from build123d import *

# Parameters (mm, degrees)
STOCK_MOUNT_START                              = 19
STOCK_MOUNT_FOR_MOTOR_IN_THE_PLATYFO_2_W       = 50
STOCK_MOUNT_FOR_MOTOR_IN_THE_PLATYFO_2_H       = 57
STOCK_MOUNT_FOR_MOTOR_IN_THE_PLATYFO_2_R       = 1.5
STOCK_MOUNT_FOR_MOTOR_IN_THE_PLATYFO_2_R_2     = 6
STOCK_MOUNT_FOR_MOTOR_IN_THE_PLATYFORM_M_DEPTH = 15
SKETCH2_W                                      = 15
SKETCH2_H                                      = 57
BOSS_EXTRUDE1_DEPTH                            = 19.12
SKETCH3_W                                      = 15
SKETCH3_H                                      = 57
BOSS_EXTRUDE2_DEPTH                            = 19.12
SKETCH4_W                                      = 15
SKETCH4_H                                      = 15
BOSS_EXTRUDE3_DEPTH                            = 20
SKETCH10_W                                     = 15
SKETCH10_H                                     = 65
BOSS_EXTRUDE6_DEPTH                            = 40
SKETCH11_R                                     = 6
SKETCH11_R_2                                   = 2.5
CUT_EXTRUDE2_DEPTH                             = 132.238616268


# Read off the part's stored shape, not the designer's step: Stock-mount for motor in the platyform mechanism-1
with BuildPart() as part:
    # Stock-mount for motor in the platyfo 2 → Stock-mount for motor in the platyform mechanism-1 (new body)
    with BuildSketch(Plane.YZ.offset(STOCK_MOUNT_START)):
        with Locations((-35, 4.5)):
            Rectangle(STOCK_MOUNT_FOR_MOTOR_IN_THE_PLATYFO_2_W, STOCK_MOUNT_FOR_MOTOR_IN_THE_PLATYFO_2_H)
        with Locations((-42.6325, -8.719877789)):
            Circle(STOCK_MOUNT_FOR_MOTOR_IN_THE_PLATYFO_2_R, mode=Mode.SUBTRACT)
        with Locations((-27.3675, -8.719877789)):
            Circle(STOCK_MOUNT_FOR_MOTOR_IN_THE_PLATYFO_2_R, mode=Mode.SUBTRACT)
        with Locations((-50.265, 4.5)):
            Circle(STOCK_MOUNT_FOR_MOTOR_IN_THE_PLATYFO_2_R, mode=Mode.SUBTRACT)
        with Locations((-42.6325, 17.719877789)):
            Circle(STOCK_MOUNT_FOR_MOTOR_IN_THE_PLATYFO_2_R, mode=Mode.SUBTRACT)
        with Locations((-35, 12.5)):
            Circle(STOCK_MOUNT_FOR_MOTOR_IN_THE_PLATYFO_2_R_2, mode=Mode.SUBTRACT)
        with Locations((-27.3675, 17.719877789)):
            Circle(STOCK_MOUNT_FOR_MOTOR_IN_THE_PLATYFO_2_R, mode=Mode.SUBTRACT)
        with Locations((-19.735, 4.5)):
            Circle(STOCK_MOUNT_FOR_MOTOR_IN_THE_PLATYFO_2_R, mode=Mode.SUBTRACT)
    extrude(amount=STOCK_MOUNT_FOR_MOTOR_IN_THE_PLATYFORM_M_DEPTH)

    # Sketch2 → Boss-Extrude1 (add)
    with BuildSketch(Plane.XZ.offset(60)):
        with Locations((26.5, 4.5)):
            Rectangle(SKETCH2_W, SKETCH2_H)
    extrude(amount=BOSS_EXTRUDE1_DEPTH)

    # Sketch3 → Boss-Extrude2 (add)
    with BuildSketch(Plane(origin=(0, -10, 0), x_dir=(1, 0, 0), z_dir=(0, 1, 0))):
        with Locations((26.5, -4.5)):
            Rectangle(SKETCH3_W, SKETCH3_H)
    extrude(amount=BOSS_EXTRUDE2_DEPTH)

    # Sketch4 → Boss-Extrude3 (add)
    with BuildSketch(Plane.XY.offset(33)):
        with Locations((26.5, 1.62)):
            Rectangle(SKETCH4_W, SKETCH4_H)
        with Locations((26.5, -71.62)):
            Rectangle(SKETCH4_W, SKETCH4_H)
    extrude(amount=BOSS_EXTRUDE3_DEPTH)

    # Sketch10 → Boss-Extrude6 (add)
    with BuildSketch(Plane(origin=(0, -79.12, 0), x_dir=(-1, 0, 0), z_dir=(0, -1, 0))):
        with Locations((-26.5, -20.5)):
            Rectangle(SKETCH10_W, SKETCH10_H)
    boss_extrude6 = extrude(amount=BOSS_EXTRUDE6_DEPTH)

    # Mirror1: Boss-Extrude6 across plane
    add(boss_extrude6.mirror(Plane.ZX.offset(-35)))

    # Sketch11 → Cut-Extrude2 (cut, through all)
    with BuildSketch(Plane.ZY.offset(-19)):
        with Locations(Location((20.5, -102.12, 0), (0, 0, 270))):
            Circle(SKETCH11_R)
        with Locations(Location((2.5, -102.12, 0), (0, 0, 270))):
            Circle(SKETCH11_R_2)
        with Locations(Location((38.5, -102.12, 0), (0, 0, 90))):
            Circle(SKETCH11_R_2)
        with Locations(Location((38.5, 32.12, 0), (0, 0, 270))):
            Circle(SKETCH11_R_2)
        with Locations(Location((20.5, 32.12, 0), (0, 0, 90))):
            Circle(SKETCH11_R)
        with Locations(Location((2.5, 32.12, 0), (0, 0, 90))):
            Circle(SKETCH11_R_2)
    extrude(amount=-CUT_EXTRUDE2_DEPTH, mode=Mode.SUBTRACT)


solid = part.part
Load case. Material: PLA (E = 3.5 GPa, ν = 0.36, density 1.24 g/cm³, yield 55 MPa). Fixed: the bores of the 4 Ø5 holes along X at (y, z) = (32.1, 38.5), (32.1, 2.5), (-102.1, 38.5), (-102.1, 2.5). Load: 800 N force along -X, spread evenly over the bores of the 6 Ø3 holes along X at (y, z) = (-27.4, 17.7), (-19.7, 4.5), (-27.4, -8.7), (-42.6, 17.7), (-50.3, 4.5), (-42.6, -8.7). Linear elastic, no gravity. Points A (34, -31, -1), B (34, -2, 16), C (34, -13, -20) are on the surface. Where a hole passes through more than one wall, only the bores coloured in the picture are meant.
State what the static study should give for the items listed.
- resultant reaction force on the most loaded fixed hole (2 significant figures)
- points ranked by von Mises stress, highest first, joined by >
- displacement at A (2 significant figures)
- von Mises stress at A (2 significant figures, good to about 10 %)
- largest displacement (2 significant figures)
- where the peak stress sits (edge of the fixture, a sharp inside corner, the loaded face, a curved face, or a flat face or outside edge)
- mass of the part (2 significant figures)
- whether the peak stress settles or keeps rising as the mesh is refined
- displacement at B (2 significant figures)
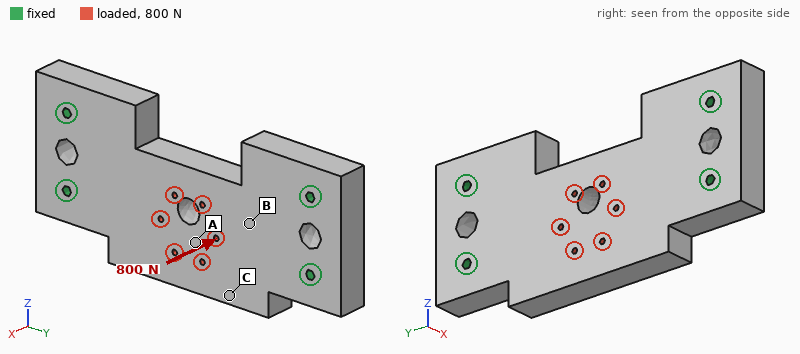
330 N
A > C > B
0.25 mm
5.4 MPa
0.30 mm
edge of the fixture
190 g
keeps rising
0.13 mm
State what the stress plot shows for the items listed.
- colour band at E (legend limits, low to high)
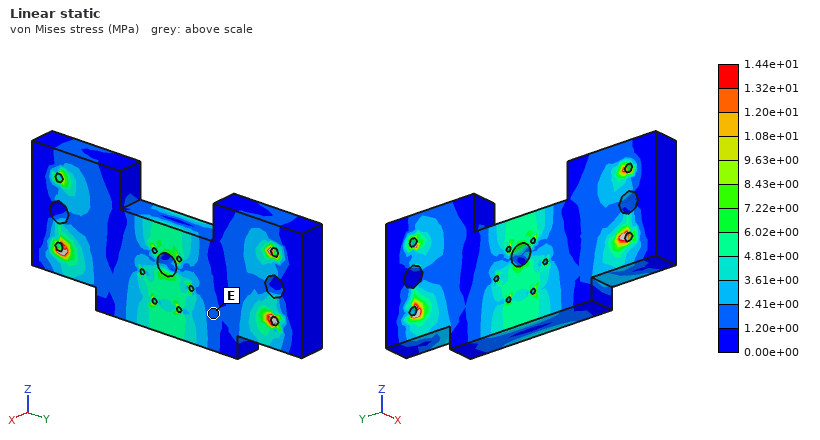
1.20e+00 to 2.41e+00 MPa
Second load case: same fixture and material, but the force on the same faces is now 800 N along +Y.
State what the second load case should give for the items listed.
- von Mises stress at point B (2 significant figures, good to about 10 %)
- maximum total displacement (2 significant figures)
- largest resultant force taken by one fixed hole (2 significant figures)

0.51 MPa
12 µm
260 N
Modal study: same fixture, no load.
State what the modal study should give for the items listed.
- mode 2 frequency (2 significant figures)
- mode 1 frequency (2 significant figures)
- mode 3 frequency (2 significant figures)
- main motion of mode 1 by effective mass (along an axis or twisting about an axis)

2000 Hz
1100 Hz
2800 Hz
along X
